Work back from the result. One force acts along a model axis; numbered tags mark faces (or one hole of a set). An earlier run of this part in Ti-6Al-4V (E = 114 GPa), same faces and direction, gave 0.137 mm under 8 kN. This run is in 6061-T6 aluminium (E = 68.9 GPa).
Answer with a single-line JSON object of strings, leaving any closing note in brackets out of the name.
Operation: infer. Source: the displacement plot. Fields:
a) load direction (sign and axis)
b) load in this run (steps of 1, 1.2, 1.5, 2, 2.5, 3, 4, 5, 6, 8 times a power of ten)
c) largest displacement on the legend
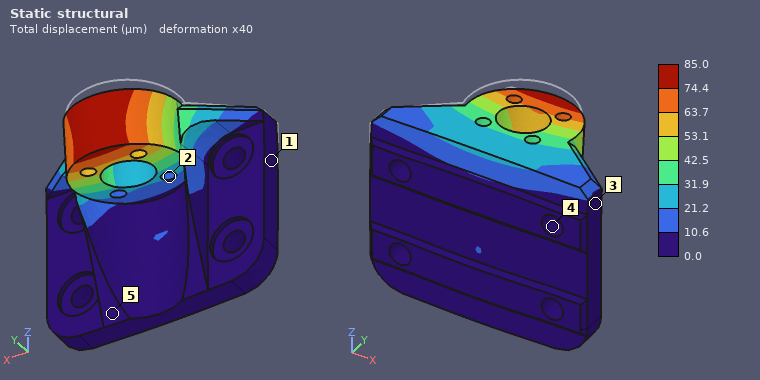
{"load direction": "-Z", "load in this run": "3 kN", "largest displacement on the legend": "85.0 µm"}
